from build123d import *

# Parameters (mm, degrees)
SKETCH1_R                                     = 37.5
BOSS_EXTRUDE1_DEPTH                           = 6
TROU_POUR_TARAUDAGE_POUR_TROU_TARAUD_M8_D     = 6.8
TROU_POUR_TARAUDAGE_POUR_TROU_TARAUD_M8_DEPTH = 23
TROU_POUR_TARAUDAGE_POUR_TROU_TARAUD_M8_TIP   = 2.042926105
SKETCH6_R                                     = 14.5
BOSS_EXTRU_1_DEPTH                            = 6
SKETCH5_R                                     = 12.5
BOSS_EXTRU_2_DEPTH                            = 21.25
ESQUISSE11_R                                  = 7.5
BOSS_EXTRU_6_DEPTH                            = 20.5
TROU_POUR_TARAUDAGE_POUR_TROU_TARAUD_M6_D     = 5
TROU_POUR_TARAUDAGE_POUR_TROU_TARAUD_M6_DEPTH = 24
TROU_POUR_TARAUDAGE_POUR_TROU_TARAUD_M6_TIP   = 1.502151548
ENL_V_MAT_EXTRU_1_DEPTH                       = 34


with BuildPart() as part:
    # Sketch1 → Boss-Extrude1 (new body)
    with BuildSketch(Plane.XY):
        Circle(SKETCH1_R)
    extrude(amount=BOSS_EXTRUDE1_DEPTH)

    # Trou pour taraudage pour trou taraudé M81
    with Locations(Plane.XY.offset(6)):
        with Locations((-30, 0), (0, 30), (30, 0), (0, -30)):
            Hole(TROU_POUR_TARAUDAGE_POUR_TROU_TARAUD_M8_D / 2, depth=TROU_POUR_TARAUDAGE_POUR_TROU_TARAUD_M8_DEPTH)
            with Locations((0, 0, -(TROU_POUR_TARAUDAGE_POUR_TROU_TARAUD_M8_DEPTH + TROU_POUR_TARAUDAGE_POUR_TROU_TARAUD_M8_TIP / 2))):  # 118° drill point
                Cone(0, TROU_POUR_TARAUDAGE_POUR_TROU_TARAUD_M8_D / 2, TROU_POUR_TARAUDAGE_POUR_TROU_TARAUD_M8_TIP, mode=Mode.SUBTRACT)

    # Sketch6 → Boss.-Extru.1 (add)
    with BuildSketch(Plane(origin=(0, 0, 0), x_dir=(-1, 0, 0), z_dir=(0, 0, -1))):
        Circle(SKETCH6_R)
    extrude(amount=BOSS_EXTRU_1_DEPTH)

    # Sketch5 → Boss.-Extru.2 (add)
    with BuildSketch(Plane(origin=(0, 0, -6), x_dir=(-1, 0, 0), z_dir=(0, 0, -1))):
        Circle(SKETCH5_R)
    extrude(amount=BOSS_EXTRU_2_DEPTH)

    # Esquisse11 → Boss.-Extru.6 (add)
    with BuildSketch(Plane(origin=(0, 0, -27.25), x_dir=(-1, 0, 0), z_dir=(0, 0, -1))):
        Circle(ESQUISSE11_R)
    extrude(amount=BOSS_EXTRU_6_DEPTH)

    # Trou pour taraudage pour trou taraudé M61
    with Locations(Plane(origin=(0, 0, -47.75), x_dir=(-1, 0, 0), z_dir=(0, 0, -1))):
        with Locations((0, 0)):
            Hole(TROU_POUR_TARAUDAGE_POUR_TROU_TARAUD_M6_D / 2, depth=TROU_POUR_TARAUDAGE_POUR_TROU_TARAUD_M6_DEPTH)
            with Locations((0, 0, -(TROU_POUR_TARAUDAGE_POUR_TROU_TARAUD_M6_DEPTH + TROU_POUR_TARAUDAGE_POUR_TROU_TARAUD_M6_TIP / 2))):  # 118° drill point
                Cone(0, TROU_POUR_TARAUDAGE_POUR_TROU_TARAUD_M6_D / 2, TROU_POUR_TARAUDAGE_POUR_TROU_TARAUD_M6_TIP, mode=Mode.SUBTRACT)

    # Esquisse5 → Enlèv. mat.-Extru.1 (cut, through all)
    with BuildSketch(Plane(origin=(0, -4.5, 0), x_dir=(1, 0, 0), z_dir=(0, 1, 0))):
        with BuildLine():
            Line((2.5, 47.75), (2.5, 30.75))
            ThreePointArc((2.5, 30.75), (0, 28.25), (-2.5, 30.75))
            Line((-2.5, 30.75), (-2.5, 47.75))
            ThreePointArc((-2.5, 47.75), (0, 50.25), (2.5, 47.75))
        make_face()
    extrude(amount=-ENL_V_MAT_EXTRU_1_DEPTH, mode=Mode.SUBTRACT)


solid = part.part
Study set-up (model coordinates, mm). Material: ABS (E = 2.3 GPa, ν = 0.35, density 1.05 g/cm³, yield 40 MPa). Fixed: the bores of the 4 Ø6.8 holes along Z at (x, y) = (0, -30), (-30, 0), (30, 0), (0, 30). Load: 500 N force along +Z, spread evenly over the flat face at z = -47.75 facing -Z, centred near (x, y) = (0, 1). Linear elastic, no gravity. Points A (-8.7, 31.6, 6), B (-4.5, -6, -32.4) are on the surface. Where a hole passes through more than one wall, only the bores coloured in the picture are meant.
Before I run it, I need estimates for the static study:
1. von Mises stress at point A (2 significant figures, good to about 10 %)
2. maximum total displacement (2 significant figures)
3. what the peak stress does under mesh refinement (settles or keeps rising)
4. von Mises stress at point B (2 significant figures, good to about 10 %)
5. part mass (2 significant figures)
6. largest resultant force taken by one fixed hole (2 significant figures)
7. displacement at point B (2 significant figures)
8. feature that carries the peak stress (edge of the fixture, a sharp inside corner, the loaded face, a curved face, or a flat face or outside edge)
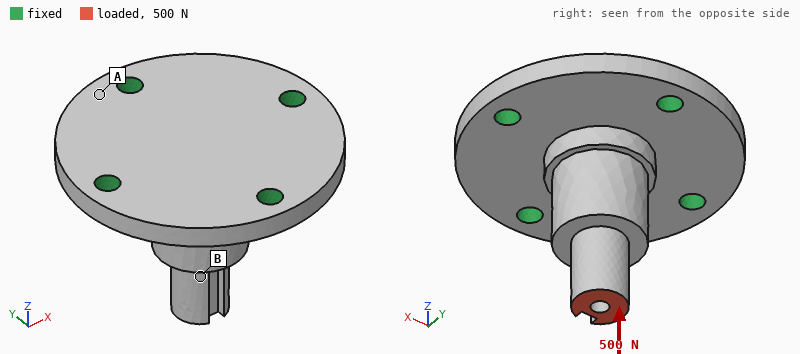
1.5 MPa
0.12 mm
keeps rising
3.4 MPa
45 g
140 N
0.091 mm
edge of the fixture
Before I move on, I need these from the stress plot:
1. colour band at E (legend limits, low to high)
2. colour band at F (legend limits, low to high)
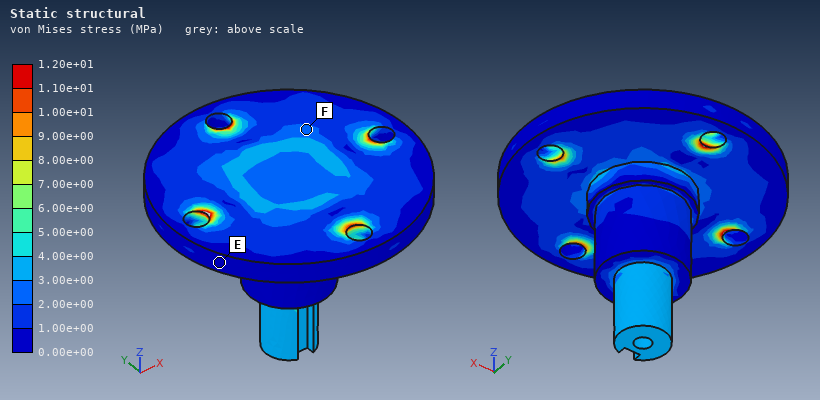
0.00e+00 to 1.00e+00 MPa
2.00e+00 to 3.00e+00 MPa
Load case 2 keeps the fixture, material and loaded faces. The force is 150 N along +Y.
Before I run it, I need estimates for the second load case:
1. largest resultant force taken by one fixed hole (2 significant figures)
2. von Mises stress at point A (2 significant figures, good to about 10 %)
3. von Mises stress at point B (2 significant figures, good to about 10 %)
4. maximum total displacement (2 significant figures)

160 N
1.1 MPa
8.4 MPa
0.48 mm
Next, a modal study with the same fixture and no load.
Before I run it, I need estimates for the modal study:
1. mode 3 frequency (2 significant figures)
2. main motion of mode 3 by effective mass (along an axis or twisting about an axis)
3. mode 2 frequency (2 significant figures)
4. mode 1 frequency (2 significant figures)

2600 Hz
along Z
1800 Hz
1800 Hz
